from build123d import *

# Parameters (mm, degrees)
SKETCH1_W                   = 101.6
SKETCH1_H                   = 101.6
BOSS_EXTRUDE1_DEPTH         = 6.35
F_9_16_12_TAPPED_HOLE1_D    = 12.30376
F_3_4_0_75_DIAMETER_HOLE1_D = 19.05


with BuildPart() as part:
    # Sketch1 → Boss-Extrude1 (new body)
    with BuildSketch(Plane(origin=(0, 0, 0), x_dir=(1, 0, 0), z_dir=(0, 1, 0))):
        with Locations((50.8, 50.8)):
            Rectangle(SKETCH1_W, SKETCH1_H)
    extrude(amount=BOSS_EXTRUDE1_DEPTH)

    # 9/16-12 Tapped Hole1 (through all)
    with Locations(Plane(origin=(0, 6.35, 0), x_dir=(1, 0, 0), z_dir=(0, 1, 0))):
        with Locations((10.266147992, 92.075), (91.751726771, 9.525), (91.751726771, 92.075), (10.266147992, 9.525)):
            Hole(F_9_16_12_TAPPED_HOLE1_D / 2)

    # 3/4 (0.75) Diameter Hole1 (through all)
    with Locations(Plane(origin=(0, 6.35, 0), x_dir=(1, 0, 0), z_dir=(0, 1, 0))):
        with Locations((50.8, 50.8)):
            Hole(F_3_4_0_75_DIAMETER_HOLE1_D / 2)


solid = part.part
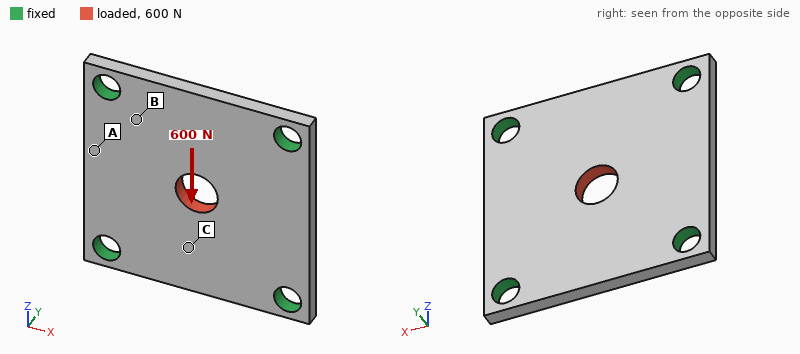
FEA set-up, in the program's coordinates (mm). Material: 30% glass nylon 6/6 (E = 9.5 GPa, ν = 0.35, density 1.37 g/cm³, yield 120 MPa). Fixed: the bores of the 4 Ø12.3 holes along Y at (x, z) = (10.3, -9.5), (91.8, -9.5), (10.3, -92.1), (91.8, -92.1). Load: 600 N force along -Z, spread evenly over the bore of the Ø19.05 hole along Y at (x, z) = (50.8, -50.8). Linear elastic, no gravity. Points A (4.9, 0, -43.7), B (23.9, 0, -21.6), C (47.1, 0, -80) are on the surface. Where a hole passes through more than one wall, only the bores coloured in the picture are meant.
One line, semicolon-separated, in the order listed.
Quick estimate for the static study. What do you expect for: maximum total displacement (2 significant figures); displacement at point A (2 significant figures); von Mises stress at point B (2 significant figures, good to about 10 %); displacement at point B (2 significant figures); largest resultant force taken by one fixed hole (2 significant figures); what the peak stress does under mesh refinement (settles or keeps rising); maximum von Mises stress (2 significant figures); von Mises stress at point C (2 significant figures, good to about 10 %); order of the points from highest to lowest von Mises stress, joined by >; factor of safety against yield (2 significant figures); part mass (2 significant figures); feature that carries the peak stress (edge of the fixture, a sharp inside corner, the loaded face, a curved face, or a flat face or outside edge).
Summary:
7.1 µm; 1.1 µm; 1.1 MPa; 2.1 µm; 170 N; settles; 2.8 MPa; 0.52 MPa; B > C > A; 44; 83 g; the loaded face
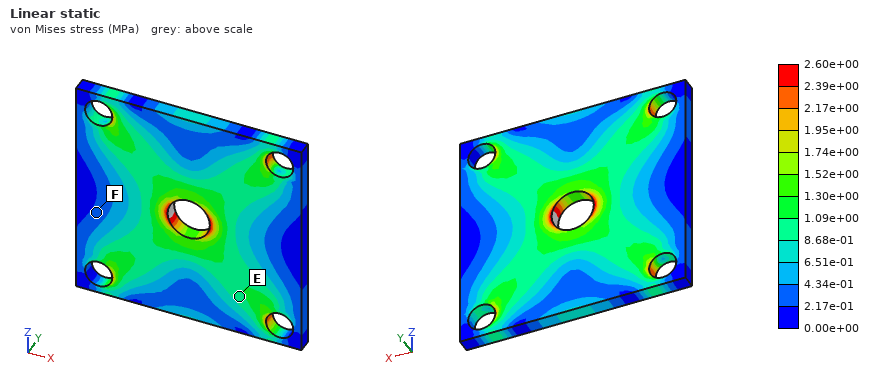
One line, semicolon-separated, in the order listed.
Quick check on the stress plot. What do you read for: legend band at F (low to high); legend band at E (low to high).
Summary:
2.17e-01 to 4.34e-01 MPa; 8.68e-01 to 1.09e+00 MPa
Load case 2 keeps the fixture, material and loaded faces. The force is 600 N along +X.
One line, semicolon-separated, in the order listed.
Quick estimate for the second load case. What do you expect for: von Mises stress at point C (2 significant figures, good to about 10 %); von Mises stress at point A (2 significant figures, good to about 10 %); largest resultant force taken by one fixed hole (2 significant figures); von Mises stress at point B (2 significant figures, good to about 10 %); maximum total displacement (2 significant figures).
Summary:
0.62 MPa; 0.42 MPa; 170 N; 1.1 MPa; 7.2 µm
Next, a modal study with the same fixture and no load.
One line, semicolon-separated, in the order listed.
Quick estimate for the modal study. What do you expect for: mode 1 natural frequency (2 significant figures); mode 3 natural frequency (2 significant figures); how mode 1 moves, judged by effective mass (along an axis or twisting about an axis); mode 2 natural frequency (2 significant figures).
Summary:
2000 Hz; 3300 Hz; along Y; 3300 Hz
